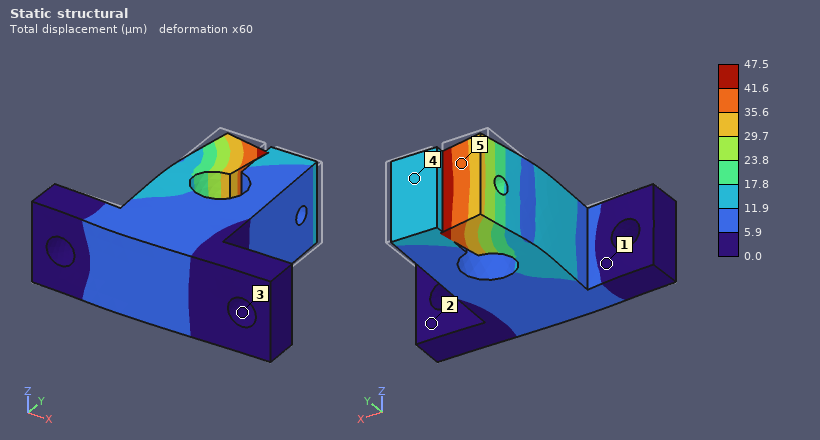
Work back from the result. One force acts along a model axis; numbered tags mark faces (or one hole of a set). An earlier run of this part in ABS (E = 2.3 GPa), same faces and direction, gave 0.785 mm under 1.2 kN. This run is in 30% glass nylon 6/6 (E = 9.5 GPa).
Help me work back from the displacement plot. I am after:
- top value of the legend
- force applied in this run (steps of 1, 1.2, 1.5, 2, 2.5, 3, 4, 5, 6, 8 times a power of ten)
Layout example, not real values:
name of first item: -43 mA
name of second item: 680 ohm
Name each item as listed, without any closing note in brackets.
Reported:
top value of the legend: 47.5 µm
force applied in this run: 300 N
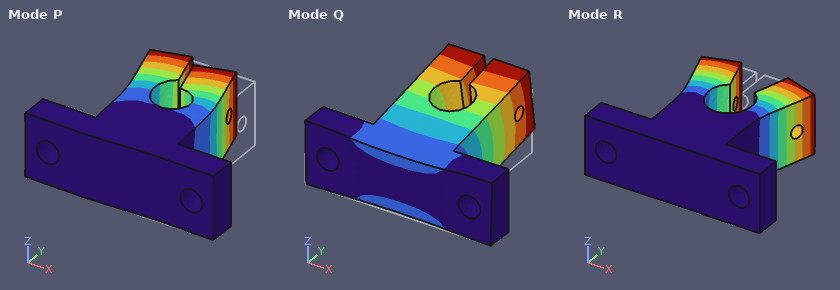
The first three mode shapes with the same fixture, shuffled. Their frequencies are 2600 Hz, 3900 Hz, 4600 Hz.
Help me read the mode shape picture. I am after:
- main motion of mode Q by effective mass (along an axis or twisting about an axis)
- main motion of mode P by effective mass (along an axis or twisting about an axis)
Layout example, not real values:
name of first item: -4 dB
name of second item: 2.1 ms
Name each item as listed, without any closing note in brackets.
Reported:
main motion of mode Q by effective mass: along Z
main motion of mode P by effective mass: along X
